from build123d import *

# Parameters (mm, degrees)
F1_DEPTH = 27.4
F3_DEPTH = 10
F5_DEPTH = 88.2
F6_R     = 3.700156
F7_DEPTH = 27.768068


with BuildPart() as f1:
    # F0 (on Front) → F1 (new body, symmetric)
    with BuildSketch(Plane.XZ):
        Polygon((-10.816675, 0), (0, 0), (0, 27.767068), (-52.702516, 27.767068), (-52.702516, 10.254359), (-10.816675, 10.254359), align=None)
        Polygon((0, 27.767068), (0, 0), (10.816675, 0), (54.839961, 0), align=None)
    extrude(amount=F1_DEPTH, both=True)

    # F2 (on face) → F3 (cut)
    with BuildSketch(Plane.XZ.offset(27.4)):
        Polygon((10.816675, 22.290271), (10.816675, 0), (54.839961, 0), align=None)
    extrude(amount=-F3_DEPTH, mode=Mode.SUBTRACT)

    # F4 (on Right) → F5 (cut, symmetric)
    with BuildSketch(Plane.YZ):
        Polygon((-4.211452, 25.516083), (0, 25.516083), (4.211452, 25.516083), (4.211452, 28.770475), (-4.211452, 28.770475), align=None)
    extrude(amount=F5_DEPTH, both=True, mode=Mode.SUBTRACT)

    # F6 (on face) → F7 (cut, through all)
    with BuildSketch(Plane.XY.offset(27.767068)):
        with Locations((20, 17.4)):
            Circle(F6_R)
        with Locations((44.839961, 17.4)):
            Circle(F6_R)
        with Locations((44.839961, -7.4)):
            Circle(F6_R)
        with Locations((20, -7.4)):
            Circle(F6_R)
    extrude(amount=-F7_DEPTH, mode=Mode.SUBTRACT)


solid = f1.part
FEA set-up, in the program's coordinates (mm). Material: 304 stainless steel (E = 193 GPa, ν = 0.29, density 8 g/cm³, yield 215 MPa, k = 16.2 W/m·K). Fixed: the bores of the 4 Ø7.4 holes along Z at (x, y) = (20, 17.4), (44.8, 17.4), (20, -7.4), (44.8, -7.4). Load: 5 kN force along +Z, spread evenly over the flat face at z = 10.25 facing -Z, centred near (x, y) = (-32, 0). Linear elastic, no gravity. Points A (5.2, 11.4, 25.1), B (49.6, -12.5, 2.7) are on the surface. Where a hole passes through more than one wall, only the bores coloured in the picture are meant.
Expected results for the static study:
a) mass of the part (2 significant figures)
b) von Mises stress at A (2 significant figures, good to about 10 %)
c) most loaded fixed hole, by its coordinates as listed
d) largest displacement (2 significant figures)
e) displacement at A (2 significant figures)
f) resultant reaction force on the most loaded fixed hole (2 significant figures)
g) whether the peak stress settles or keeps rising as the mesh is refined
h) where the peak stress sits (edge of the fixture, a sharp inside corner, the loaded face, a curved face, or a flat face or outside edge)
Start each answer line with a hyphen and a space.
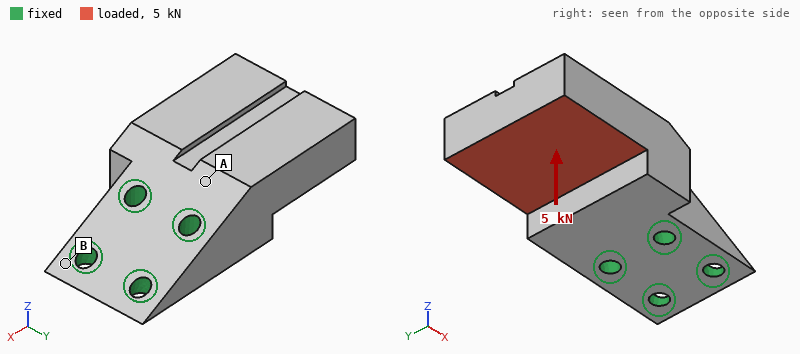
- 720 g
- 31 MPa
- (20, -7.4)
- 67 µm
- 11 µm
- 3.3 kN
- keeps rising
- edge of the fixture
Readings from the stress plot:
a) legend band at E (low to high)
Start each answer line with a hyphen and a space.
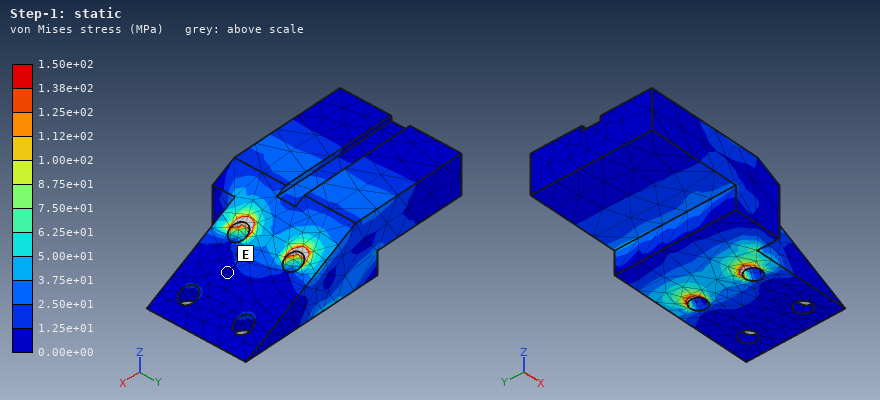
- 0.00e+00 to 1.25e+01 MPa
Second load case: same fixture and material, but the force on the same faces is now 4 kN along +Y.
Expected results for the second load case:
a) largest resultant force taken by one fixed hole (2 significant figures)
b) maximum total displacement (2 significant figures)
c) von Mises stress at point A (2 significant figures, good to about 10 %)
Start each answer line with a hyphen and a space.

- 6.9 kN
- 19 µm
- 5.8 MPa
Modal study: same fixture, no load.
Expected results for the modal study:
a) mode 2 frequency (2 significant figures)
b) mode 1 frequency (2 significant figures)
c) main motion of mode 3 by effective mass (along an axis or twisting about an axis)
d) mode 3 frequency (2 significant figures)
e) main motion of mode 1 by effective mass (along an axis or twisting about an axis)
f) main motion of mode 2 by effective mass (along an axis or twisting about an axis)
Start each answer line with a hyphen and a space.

- 5000 Hz
- 2900 Hz
- twisting about X
- 6900 Hz
- along Z
- along Y
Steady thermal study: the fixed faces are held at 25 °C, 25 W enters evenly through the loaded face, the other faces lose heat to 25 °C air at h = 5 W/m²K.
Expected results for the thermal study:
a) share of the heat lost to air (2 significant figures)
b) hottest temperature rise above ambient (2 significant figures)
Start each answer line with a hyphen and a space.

- 9.0 %
- 77 K
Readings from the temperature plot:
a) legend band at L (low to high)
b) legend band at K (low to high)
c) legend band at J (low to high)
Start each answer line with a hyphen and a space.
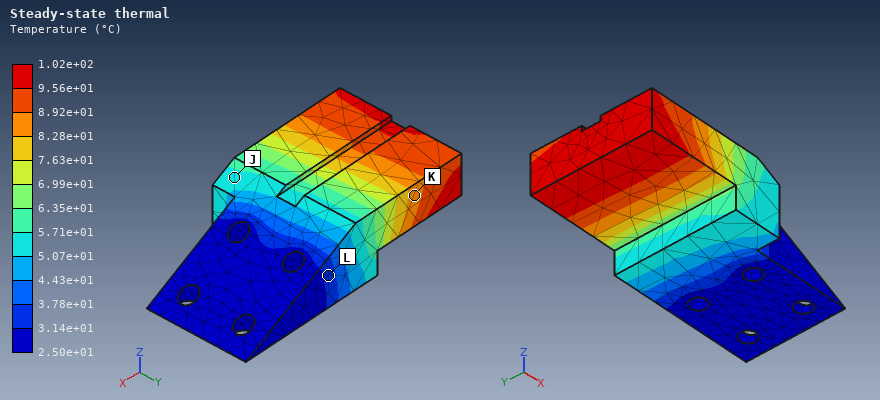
- 3.14e+01 to 3.78e+01 °C
- 8.28e+01 to 8.92e+01 °C
- 5.07e+01 to 5.71e+01 °C
